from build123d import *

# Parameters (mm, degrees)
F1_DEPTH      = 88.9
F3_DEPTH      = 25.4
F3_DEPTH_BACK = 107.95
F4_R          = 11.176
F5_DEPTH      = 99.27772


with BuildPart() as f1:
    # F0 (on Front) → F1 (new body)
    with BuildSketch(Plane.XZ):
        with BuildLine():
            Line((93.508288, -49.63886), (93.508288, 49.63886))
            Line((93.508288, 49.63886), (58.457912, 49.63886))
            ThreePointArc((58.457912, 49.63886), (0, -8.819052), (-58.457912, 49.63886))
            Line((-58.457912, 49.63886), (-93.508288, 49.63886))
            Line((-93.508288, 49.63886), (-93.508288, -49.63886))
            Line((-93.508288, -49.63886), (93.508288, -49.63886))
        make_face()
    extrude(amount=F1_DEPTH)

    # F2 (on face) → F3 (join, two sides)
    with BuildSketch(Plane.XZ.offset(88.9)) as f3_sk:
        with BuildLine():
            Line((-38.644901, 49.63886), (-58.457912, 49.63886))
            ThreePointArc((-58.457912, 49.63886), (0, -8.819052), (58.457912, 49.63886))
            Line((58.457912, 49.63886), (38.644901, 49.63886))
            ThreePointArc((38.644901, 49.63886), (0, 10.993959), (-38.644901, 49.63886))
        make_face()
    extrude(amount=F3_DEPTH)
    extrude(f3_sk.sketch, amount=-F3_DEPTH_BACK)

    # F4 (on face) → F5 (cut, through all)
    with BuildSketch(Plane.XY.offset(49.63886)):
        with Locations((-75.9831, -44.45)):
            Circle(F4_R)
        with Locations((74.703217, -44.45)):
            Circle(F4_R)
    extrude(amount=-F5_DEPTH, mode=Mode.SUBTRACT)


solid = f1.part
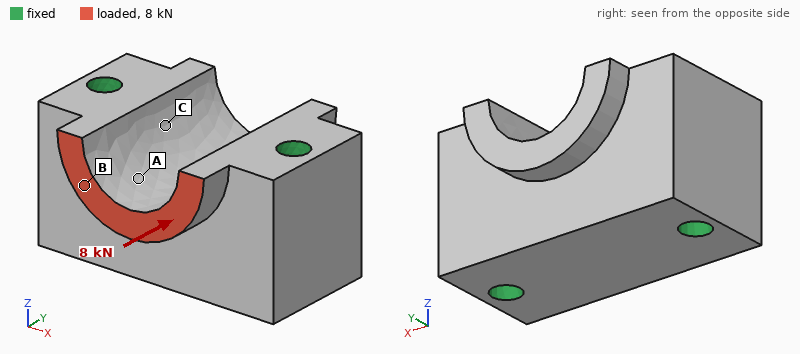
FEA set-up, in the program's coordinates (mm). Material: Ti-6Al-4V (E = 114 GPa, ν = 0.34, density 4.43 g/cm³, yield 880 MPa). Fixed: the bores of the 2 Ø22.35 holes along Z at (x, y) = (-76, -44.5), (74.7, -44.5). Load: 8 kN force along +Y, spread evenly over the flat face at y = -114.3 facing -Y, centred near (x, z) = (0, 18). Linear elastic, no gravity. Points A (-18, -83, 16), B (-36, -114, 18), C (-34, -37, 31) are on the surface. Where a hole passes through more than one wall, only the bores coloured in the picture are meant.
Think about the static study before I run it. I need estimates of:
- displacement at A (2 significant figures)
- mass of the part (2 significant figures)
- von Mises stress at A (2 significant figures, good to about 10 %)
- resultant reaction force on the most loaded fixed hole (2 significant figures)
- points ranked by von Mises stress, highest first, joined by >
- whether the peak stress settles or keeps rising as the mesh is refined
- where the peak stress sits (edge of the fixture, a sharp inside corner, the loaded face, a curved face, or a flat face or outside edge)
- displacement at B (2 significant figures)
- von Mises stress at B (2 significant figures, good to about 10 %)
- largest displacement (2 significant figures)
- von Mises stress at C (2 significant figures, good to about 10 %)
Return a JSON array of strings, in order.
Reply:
["1.2 µm", "6.6 kg", "1.5 MPa", "4.1 kN", "B > A > C", "keeps rising", "edge of the fixture", "1.8 µm", "2.6 MPa", "2.6 µm", "0.73 MPa"]
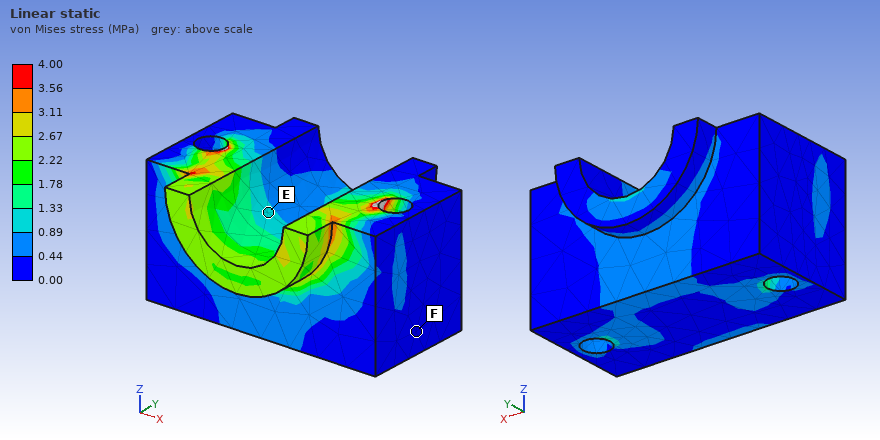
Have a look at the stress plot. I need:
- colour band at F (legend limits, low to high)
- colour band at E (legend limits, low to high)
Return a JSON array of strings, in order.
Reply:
["0.00 to 0.44 MPa", "0.89 to 1.33 MPa"]
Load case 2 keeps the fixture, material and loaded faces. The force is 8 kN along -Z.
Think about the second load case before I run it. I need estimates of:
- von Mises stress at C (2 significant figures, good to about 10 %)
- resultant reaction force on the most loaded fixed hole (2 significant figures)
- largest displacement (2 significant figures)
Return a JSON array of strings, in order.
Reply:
["0.95 MPa", "4.1 kN", "10 µm"]
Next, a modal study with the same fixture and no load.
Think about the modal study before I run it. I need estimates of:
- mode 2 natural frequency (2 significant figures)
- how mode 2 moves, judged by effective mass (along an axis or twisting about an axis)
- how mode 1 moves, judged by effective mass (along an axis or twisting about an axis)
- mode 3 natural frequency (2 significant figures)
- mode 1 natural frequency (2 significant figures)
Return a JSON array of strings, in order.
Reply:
["8300 Hz", "along Z", "along Y", "9100 Hz", "7500 Hz"]
